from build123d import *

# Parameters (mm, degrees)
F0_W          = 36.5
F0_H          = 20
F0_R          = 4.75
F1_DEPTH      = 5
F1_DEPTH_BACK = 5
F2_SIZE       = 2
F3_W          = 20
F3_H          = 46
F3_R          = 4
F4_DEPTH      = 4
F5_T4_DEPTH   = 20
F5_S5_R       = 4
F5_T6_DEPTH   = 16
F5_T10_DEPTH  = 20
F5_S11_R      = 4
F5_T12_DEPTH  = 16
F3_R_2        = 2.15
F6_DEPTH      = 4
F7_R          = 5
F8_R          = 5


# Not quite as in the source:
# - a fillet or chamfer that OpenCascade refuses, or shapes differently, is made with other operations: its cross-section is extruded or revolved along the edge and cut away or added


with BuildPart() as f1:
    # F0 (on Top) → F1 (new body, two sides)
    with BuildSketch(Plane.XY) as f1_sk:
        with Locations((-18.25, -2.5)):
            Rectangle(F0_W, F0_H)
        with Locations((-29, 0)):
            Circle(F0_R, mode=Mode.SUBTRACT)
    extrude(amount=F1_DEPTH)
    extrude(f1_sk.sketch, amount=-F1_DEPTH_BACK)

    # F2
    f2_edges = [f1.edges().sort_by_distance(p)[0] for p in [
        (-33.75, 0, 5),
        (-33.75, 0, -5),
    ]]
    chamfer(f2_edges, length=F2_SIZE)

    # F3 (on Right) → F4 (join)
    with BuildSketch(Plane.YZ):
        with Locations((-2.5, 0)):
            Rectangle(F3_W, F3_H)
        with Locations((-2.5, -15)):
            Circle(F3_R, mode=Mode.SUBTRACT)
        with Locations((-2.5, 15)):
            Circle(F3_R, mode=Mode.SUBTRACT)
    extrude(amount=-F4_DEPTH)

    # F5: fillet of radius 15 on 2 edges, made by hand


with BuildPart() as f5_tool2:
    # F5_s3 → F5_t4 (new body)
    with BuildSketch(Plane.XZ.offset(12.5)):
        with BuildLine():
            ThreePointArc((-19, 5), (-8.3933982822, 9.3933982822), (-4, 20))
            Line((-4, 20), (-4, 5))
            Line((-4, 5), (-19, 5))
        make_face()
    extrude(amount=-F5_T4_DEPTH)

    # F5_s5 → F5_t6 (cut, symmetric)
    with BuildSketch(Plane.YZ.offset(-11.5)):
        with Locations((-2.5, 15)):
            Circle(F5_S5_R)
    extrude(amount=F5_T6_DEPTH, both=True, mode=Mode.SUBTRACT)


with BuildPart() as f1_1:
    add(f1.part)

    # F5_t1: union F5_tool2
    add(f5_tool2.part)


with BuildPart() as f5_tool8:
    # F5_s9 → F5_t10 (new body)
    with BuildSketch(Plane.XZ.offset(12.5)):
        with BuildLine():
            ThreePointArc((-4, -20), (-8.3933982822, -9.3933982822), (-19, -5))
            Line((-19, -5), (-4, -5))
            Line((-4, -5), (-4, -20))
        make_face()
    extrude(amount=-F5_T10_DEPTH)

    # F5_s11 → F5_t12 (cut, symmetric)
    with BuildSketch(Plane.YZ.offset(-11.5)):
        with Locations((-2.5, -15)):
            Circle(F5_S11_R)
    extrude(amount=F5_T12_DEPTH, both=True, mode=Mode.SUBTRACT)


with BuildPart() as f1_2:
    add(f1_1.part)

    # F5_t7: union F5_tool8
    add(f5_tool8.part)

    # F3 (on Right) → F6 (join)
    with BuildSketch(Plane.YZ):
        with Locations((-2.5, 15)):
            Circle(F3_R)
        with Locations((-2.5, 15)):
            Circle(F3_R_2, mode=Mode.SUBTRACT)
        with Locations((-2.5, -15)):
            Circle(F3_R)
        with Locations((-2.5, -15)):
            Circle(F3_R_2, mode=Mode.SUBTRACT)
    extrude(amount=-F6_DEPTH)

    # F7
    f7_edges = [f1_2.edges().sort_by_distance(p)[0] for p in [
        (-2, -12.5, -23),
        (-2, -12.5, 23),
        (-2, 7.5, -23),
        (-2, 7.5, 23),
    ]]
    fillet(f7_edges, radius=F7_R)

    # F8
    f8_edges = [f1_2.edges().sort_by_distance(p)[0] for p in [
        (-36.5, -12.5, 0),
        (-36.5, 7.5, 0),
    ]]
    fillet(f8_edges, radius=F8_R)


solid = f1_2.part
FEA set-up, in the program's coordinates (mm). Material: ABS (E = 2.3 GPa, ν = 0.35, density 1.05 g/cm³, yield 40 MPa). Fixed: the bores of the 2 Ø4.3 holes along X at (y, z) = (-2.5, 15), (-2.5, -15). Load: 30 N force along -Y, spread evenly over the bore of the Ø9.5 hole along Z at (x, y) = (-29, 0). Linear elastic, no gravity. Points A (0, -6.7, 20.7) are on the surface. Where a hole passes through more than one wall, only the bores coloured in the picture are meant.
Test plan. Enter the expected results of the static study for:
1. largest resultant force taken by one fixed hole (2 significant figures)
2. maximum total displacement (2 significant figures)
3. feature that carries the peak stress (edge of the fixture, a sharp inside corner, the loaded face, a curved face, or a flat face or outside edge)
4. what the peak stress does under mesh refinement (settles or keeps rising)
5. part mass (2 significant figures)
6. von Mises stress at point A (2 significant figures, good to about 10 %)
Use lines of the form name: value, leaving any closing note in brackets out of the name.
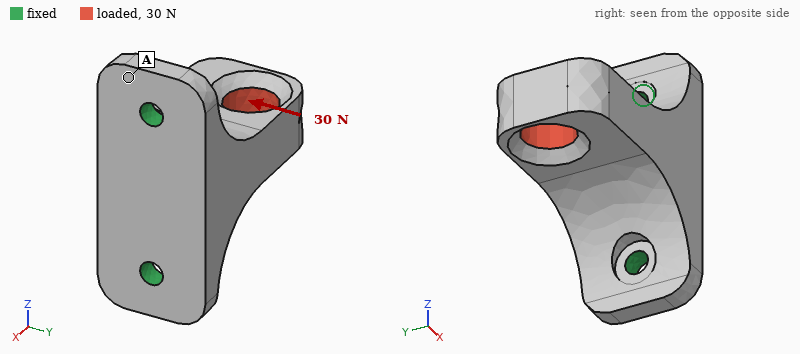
largest resultant force taken by one fixed hole: 15 N
maximum total displacement: 0.16 mm
feature that carries the peak stress: edge of the fixture
what the peak stress does under mesh refinement: keeps rising
part mass: 11 g
von Mises stress at point A: 1.2 MPa
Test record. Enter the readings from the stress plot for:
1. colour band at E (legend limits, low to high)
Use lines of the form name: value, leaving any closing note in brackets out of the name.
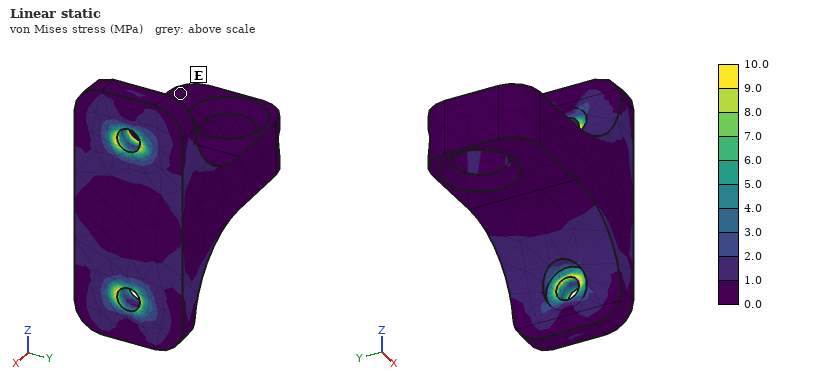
colour band at E: 0.0 to 1.0 MPa
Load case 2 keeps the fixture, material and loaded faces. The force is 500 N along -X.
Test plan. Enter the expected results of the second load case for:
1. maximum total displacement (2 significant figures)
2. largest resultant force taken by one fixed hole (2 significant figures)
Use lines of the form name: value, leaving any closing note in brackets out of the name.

maximum total displacement: 0.30 mm
largest resultant force taken by one fixed hole: 290 N
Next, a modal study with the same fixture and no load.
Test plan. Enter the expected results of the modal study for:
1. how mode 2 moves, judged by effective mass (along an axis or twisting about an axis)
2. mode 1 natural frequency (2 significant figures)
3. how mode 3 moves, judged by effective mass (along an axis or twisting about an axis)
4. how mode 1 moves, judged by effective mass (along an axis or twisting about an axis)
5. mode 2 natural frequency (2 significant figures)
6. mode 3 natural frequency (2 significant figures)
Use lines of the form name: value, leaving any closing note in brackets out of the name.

how mode 2 moves, judged by effective mass: along Z
mode 1 natural frequency: 1300 Hz
how mode 3 moves, judged by effective mass: along X
how mode 1 moves, judged by effective mass: along Y
mode 2 natural frequency: 3100 Hz
mode 3 natural frequency: 5100 Hz
